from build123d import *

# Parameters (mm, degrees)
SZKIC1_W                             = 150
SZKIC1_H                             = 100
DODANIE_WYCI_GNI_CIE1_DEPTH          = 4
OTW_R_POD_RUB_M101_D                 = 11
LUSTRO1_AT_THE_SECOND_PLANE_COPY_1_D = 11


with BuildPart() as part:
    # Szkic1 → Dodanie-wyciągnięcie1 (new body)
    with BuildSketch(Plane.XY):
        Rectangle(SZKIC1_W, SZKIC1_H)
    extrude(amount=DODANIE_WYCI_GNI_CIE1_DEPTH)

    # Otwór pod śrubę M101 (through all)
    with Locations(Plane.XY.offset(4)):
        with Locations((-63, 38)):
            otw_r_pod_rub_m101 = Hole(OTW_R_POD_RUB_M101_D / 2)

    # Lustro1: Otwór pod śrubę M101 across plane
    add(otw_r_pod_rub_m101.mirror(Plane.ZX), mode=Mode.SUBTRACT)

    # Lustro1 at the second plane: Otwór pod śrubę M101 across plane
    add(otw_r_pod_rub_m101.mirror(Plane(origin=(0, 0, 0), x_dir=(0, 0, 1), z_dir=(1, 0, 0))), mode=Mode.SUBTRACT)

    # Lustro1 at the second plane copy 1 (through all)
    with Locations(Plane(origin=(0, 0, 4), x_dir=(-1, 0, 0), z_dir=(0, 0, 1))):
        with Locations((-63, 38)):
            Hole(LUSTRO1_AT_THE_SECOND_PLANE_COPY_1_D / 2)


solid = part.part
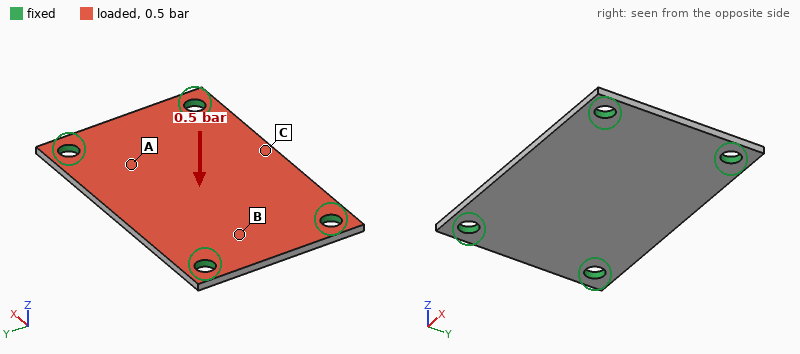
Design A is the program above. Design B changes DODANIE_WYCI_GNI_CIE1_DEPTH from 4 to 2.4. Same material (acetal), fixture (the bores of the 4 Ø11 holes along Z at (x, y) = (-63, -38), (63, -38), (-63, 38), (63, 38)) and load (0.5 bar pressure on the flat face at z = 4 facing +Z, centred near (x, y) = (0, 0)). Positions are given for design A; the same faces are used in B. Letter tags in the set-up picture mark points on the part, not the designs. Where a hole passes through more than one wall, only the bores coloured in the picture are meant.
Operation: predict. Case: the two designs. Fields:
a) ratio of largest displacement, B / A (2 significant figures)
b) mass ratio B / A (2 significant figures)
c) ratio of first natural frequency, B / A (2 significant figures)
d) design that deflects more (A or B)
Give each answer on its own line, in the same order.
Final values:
4.5
0.60
0.61
B
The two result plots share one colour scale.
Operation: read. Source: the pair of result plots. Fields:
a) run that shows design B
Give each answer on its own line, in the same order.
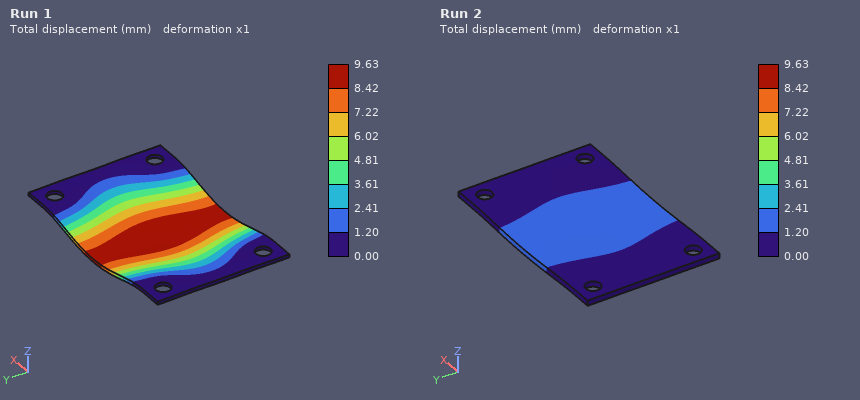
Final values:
Run 1
